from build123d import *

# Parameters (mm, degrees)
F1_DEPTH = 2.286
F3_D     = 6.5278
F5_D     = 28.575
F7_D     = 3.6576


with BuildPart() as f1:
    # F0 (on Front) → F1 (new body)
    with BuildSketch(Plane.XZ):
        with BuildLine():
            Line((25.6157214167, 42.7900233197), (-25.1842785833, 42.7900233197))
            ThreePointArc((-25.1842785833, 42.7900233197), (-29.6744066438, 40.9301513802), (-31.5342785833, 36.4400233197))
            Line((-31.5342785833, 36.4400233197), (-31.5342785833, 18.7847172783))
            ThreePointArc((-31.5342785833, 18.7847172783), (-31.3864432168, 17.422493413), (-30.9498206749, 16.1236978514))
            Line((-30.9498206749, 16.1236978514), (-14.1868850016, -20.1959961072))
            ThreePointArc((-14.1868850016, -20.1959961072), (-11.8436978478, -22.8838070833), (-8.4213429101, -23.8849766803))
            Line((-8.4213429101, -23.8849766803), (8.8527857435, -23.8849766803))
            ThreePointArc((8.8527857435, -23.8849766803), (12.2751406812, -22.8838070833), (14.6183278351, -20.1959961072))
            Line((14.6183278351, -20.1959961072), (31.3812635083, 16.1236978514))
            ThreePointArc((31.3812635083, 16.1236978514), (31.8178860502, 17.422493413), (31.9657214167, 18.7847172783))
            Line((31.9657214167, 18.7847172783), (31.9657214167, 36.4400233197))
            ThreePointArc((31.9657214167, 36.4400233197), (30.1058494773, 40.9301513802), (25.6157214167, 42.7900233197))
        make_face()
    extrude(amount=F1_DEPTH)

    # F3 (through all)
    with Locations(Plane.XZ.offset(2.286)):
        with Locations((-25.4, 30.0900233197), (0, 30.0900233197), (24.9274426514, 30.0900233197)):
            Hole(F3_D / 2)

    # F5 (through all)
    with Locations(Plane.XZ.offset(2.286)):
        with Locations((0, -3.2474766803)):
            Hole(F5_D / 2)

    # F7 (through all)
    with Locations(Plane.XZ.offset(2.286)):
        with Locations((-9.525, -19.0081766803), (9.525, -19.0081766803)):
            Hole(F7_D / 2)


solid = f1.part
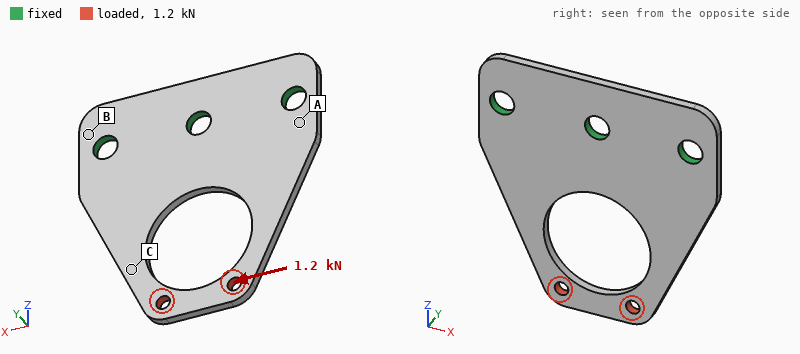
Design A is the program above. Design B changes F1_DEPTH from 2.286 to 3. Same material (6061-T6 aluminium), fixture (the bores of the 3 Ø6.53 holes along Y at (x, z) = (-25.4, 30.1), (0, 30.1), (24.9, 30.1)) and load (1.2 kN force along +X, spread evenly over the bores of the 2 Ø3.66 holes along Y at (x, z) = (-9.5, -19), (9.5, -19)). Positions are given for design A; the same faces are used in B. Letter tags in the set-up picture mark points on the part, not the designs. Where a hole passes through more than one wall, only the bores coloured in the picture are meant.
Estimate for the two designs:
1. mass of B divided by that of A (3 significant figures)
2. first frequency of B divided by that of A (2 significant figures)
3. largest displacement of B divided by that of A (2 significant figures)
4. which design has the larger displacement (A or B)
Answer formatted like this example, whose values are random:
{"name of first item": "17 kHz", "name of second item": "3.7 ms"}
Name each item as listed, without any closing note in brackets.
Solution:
{"mass of B divided by that of A": "1.31", "first frequency of B divided by that of A": "1.3", "largest displacement of B divided by that of A": "0.76", "which design has the larger displacement": "A"}
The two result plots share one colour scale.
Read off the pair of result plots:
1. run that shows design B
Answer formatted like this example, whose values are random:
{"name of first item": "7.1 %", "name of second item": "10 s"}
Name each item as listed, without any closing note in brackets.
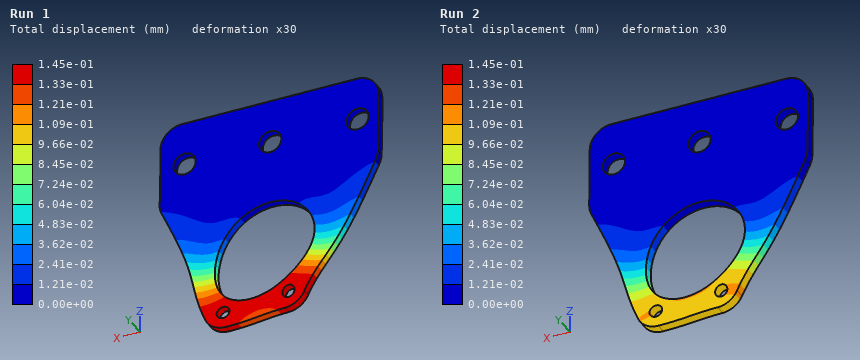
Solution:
{"run that shows design B": "Run 2"}
